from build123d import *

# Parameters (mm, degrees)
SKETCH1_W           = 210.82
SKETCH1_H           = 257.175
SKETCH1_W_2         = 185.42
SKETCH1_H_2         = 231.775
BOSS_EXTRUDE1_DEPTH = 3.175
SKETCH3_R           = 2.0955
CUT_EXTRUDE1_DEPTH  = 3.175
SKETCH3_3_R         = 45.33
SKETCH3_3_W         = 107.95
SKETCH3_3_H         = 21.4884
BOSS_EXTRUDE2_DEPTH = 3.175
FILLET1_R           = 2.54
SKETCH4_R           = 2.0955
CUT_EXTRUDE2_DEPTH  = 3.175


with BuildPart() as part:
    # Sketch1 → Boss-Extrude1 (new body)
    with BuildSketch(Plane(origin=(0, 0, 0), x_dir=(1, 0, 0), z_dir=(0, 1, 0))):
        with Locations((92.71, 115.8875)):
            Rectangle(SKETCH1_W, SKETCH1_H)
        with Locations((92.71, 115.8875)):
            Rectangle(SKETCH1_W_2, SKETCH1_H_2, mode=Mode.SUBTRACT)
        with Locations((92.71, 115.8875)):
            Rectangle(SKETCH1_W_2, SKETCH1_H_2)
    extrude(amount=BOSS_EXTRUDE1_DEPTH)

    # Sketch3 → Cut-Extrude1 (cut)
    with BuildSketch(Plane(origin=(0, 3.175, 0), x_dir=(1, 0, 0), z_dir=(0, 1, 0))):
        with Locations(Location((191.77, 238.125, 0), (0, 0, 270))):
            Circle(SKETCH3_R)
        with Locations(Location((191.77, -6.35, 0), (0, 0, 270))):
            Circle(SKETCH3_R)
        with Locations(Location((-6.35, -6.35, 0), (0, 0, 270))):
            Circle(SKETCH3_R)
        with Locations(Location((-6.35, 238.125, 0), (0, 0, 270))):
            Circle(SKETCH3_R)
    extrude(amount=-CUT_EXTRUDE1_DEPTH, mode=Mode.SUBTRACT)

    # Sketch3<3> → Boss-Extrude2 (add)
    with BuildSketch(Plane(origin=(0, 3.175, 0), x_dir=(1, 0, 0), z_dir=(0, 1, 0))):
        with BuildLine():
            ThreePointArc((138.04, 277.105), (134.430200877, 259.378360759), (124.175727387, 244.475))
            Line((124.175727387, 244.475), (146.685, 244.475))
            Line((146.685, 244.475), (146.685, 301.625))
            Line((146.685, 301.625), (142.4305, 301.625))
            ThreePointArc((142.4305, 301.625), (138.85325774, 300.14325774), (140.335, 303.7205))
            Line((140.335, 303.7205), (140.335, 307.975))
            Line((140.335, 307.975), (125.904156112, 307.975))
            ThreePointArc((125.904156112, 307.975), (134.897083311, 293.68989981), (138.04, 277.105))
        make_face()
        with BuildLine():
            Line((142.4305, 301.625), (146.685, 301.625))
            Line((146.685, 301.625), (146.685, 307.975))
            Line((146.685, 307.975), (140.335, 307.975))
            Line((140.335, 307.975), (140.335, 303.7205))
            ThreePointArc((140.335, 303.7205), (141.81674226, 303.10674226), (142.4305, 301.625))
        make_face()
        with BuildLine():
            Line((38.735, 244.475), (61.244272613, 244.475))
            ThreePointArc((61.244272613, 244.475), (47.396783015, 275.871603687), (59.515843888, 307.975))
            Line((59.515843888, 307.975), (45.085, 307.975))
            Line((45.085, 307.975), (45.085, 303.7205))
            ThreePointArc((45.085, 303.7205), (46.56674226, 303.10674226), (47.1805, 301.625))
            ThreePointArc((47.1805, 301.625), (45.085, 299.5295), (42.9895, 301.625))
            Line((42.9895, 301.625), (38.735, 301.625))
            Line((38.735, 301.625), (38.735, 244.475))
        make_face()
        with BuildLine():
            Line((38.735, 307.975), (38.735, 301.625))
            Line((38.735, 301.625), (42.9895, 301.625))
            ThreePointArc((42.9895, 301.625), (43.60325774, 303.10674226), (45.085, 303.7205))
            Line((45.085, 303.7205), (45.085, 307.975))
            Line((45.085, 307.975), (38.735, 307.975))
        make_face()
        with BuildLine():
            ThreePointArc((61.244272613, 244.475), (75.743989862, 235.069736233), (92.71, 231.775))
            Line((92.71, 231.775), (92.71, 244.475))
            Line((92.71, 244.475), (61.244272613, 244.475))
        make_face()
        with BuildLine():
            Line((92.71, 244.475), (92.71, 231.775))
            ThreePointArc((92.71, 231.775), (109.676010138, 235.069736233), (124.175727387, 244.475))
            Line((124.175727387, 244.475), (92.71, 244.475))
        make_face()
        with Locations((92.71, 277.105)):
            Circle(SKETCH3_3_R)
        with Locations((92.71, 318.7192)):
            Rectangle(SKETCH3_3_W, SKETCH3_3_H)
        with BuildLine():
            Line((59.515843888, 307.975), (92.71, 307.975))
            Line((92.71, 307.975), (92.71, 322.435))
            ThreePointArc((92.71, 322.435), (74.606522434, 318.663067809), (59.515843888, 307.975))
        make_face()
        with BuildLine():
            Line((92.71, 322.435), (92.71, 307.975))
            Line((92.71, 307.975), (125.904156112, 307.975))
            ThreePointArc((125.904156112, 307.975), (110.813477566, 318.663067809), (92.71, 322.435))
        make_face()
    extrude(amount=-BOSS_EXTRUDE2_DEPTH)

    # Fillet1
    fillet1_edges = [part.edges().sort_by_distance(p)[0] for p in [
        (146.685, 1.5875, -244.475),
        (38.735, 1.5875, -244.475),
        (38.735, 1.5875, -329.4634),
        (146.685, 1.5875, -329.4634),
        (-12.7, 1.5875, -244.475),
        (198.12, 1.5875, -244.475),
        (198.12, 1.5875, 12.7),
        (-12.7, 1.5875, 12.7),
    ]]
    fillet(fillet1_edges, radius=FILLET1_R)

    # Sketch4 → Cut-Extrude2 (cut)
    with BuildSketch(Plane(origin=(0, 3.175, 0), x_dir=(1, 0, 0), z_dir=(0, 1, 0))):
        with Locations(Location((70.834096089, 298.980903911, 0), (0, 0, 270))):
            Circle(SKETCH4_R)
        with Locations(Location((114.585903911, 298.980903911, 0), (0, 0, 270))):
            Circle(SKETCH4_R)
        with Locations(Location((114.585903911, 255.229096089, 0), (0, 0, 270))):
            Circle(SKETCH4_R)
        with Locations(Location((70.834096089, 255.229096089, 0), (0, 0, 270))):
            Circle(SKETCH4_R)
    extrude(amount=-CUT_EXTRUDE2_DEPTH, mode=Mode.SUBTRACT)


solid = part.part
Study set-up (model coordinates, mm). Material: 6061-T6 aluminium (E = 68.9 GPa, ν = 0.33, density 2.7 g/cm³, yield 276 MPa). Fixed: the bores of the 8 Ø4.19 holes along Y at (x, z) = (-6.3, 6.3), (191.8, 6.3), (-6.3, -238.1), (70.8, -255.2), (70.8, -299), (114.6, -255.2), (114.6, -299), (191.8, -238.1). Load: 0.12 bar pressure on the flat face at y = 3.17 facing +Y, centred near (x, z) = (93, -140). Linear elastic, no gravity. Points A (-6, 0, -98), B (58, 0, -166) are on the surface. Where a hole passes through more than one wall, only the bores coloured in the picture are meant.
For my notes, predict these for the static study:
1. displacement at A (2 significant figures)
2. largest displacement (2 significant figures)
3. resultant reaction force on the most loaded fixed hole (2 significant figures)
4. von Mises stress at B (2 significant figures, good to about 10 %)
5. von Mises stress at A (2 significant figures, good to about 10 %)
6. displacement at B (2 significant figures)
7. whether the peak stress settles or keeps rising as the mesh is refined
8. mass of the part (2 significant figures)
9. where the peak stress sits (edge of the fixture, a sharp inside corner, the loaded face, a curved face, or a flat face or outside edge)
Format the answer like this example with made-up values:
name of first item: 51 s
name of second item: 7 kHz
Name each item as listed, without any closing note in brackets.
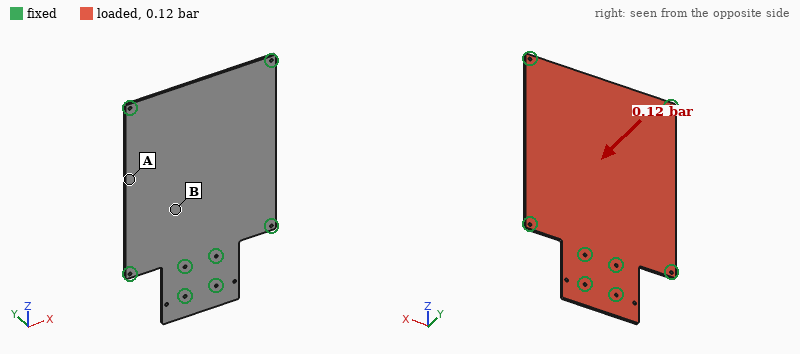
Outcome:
displacement at A: 1.0 mm
largest displacement: 1.2 mm
resultant reaction force on the most loaded fixed hole: 150 N
von Mises stress at B: 12 MPa
von Mises stress at A: 27 MPa
displacement at B: 0.83 mm
whether the peak stress settles or keeps rising as the mesh is refined: keeps rising
mass of the part: 540 g
where the peak stress sits: edge of the fixture
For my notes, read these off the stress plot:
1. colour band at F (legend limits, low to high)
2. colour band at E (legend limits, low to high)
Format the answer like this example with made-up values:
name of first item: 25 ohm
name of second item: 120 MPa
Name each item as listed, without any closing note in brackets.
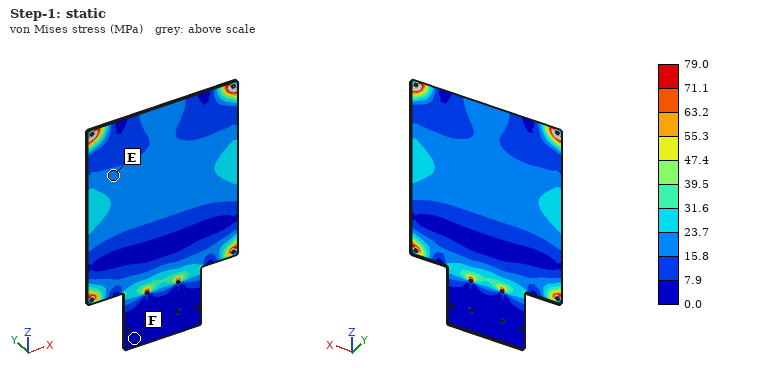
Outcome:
colour band at F: 0.0 to 7.9 MPa
colour band at E: 15.8 to 23.7 MPa
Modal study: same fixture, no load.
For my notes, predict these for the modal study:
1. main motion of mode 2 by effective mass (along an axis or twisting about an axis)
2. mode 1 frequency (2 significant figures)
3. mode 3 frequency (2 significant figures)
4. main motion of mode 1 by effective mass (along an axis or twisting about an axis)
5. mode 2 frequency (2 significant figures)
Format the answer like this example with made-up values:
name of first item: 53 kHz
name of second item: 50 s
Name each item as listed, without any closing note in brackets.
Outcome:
main motion of mode 2 by effective mass: twisting about Z
mode 1 frequency: 200 Hz
mode 3 frequency: 410 Hz
main motion of mode 1 by effective mass: along Y
mode 2 frequency: 320 Hz
